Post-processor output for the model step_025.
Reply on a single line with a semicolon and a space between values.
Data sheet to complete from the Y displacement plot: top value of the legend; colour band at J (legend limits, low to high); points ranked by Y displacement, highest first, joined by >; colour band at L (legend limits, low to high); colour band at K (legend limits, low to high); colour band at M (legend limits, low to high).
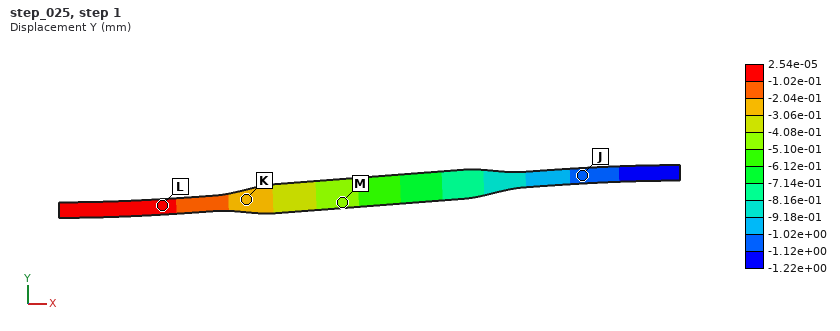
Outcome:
2.54e-05 mm; -1.12e+00 to -1.02e+00 mm; L > K > M > J; -1.02e-01 to 2.54e-05 mm; -3.06e-01 to -2.04e-01 mm; -5.10e-01 to -4.08e-01 mm
